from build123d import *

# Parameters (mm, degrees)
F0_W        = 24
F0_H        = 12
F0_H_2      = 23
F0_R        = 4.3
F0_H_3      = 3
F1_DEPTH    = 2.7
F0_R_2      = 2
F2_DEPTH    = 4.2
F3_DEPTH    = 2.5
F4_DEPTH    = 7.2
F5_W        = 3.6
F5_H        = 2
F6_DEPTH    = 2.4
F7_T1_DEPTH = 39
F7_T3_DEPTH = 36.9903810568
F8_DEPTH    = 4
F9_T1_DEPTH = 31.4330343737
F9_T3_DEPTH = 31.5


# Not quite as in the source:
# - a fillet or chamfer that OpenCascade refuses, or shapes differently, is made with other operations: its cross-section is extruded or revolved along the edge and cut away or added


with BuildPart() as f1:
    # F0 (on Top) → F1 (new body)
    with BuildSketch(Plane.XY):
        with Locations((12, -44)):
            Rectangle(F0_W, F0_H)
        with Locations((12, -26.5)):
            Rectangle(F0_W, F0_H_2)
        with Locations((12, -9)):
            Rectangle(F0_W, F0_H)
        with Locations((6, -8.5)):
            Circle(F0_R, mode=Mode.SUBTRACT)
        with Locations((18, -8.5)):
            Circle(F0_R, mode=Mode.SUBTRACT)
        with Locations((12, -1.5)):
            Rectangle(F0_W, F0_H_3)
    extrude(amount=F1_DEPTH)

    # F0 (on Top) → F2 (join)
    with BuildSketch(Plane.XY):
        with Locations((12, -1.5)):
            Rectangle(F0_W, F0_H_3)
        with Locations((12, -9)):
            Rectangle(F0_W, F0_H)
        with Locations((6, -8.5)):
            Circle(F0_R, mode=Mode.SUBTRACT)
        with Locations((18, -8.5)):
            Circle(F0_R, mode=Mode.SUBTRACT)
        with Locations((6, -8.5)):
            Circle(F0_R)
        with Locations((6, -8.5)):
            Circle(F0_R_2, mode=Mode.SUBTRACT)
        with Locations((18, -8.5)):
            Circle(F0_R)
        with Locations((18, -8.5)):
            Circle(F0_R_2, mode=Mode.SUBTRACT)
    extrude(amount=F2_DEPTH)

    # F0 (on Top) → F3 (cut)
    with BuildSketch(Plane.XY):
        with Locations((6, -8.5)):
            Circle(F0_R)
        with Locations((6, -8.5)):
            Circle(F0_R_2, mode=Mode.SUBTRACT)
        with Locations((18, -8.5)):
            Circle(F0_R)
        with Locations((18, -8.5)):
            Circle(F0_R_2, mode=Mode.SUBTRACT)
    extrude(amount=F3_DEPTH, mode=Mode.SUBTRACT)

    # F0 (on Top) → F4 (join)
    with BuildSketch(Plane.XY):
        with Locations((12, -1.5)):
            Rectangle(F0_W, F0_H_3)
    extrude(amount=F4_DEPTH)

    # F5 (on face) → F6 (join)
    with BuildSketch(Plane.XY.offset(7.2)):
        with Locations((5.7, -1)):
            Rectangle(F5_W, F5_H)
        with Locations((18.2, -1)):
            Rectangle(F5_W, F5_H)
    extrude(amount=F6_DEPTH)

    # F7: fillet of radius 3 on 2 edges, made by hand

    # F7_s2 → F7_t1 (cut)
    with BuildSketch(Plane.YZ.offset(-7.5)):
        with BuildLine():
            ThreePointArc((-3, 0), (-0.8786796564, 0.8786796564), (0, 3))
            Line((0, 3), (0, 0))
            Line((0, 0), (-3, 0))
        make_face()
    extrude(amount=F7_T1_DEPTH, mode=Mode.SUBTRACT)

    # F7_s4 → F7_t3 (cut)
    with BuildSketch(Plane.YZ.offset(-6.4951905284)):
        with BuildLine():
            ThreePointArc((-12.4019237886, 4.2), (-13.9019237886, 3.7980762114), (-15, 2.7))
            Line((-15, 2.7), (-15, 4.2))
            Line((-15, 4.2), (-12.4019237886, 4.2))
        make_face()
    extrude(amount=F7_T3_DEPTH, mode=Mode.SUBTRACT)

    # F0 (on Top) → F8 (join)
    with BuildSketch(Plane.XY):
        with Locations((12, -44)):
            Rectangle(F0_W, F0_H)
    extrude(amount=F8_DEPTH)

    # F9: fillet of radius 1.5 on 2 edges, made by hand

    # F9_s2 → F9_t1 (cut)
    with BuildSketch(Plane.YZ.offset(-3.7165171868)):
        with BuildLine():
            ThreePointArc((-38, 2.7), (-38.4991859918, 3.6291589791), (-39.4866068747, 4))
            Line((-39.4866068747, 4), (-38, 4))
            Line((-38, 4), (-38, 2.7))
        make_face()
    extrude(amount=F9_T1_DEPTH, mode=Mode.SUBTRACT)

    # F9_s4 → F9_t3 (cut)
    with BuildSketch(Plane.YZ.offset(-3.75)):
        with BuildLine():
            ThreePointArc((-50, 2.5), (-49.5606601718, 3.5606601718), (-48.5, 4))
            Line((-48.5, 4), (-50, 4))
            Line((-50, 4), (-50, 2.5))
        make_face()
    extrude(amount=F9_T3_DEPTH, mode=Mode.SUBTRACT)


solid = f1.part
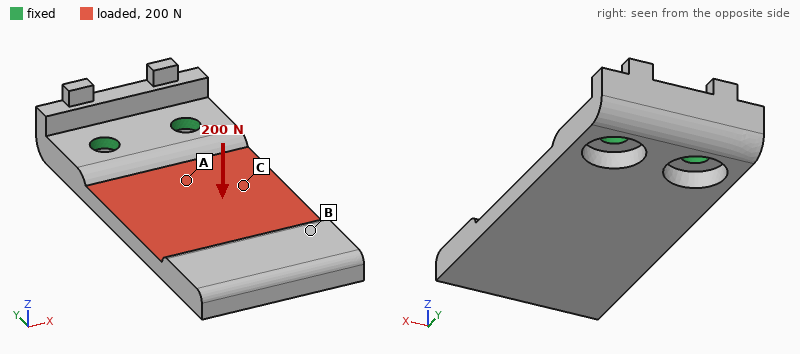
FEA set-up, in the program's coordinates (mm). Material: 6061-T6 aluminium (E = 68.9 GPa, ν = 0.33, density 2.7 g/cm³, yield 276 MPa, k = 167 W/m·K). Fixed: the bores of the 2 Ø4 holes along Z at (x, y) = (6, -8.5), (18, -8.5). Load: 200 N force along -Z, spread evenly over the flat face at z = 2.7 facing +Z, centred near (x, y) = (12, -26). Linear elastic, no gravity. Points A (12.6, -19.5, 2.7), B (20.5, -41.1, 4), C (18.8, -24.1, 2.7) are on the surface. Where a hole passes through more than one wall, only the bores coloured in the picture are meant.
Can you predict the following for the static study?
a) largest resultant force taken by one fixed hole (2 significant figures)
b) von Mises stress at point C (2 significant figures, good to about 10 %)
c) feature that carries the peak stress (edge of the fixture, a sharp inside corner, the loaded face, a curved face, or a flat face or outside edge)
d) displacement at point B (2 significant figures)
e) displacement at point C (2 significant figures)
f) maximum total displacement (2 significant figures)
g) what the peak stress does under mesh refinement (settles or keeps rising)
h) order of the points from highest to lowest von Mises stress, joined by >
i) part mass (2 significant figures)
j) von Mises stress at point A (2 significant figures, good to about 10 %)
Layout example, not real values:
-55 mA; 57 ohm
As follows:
110 N; 28 MPa; edge of the fixture; 0.30 mm; 0.099 mm; 0.40 mm; keeps rising; A > C > B; 11 g; 46 MPa
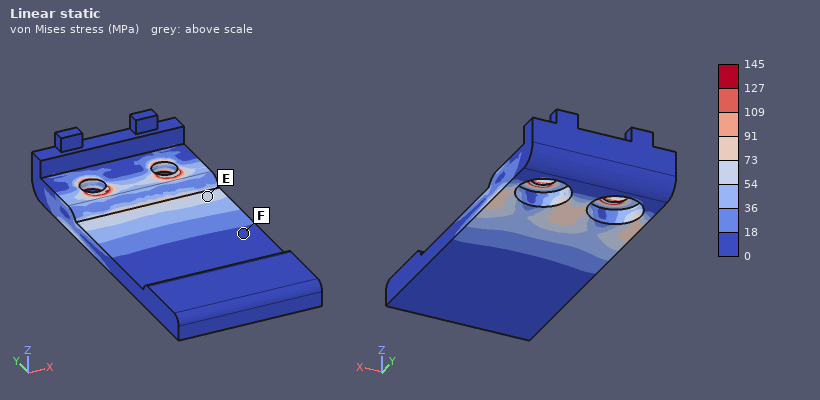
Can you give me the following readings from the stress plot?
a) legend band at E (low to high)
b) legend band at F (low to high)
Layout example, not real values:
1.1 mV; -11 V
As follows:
54 to 73 MPa; 0 to 18 MPa
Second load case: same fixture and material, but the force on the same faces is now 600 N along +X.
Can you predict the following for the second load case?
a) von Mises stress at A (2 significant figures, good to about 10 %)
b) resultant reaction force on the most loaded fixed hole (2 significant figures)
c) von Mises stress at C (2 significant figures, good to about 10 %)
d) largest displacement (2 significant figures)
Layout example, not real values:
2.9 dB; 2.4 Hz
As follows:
40 MPa; 760 N; 29 MPa; 70 µm
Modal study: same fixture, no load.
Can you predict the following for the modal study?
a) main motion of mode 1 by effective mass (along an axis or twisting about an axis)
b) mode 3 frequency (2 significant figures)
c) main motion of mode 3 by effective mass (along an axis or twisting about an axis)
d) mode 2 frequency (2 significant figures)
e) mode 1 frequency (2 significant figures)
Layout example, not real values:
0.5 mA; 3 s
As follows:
along Z; 6800 Hz; along X; 4300 Hz; 1200 Hz
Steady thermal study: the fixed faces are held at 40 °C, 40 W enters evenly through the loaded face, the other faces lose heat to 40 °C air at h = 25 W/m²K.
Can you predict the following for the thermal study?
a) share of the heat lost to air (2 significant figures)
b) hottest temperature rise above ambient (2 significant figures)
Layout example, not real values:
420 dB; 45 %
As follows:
5.8 %; 64 K
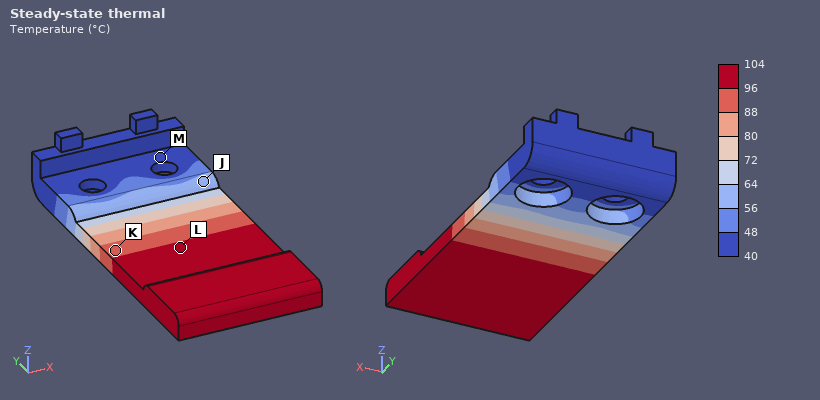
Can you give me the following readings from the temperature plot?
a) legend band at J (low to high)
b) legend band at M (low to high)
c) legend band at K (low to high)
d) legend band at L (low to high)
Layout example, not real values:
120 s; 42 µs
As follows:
56 to 64 °C; 40 to 48 °C; 88 to 96 °C; 96 to 104 °C
